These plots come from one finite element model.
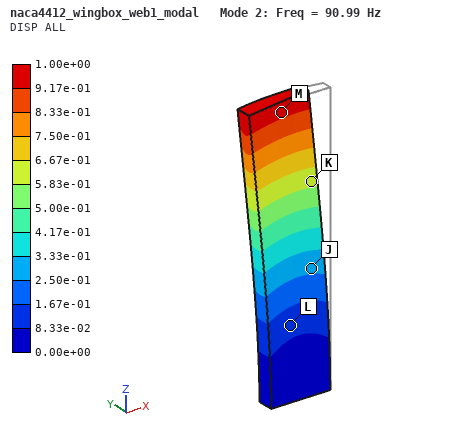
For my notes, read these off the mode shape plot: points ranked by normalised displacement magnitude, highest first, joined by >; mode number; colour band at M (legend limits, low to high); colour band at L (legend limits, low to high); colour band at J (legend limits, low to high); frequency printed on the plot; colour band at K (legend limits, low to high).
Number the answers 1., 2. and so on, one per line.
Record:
1. M > K > J > L
2. 2
3. 9.17e-01 to 1.00e+00
4. 8.33e-02 to 1.67e-01
5. 2.50e-01 to 3.33e-01
6. 90.99 Hz
7. 5.83e-01 to 6.67e-01
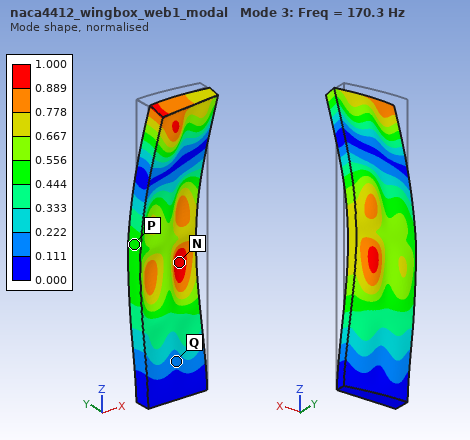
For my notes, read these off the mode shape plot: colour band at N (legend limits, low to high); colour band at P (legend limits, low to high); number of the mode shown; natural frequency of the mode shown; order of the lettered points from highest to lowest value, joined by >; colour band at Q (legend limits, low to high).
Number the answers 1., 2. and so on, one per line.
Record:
1. 0.889 to 1.000
2. 0.444 to 0.556
3. 3
4. 170.3 Hz
5. N > P > Q
6. 0.111 to 0.222
